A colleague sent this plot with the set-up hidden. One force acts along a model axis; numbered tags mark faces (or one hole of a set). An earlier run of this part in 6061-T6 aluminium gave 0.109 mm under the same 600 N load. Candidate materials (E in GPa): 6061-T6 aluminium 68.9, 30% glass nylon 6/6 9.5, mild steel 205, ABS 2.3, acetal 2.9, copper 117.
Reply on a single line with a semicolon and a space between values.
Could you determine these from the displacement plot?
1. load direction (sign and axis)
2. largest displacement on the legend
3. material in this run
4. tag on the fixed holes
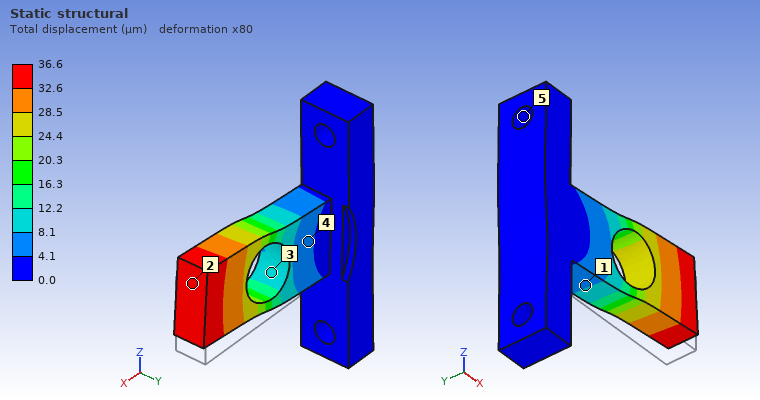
+Z; 36.6 µm; mild steel; 5
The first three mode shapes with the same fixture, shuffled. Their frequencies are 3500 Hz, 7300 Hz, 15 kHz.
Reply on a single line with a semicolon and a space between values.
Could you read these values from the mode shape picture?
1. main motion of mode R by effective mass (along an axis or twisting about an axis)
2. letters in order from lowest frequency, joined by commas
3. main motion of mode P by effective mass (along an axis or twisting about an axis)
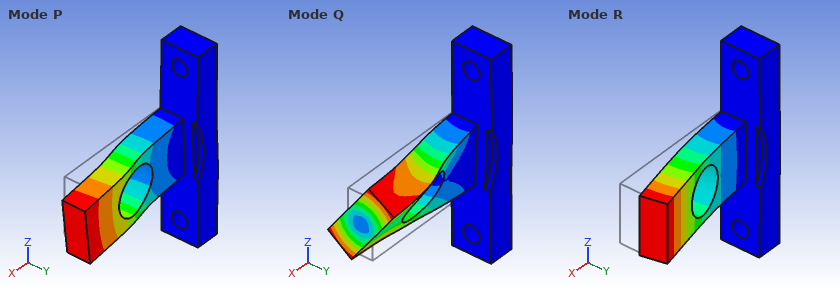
along Y; R, P, Q; along Z
